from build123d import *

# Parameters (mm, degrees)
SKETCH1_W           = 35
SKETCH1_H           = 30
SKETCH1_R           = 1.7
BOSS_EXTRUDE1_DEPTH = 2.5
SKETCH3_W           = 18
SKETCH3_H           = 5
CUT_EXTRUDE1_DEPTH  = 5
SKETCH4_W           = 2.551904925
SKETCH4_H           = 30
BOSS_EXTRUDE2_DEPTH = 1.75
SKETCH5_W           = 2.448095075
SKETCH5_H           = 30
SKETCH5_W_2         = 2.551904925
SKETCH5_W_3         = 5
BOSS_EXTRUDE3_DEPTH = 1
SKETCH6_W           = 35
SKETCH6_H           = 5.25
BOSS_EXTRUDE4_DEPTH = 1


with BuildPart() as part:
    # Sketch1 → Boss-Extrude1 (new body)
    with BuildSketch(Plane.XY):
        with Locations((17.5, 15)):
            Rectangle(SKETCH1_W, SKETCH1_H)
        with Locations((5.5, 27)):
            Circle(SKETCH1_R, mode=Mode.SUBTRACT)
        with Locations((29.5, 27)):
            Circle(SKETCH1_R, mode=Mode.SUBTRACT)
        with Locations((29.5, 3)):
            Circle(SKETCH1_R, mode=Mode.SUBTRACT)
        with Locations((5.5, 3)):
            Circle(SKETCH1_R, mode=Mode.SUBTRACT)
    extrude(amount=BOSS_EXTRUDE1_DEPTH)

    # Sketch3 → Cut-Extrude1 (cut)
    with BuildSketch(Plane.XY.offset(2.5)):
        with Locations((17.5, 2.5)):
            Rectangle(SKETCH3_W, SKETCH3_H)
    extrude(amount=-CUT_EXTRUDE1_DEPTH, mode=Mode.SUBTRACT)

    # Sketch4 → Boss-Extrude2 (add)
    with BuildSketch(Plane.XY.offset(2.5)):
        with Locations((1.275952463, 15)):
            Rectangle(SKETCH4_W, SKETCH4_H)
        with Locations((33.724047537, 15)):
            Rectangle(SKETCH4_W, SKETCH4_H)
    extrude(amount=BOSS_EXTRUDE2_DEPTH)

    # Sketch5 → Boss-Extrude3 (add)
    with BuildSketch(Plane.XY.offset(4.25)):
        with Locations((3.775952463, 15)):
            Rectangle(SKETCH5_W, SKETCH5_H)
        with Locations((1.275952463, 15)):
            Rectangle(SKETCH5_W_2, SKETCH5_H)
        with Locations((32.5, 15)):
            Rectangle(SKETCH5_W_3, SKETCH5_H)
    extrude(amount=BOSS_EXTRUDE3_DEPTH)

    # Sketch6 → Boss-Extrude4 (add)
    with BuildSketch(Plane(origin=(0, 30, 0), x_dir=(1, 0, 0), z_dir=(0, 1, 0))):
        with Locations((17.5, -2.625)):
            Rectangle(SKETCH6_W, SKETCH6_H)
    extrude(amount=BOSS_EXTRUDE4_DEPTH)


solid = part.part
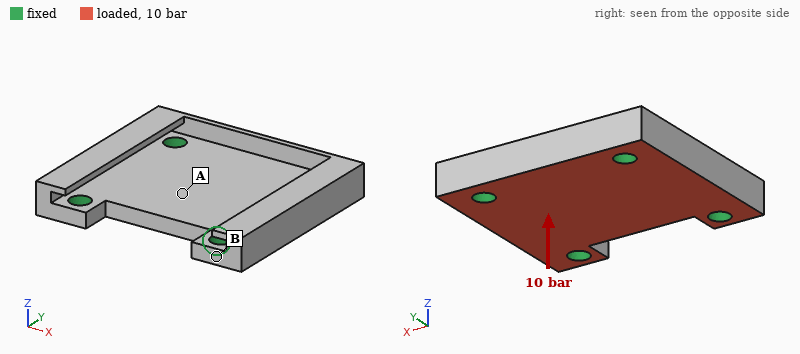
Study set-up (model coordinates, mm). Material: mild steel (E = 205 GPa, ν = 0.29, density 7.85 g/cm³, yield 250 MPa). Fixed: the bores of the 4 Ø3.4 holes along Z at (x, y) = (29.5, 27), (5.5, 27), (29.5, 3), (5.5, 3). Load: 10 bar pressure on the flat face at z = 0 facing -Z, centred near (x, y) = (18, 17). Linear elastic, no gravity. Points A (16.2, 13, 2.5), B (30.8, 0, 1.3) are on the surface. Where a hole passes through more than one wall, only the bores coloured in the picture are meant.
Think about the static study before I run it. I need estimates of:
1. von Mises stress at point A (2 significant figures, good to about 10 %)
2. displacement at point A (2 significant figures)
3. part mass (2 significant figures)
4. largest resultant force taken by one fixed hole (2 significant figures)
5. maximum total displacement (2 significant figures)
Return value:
24 MPa
6.5 µm
24 g
270 N
6.6 µm
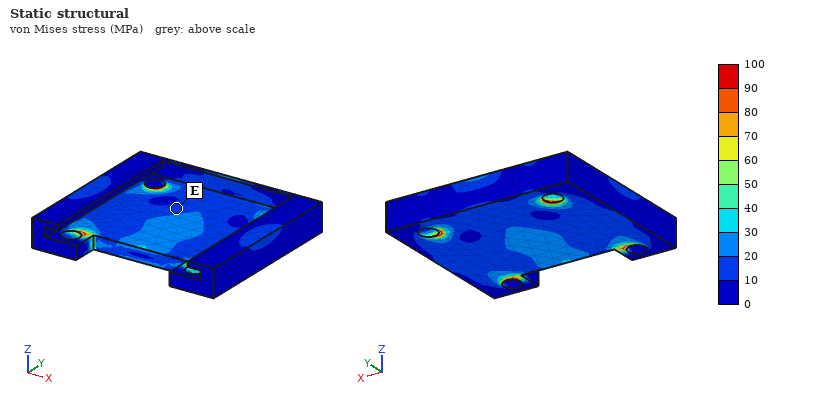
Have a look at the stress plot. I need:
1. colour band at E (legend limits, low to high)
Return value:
10 to 20 MPa
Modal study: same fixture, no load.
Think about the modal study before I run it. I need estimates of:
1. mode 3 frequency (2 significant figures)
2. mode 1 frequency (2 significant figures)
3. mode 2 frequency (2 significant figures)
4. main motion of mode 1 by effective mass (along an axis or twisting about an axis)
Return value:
27 kHz
17 kHz
27 kHz
along Z
